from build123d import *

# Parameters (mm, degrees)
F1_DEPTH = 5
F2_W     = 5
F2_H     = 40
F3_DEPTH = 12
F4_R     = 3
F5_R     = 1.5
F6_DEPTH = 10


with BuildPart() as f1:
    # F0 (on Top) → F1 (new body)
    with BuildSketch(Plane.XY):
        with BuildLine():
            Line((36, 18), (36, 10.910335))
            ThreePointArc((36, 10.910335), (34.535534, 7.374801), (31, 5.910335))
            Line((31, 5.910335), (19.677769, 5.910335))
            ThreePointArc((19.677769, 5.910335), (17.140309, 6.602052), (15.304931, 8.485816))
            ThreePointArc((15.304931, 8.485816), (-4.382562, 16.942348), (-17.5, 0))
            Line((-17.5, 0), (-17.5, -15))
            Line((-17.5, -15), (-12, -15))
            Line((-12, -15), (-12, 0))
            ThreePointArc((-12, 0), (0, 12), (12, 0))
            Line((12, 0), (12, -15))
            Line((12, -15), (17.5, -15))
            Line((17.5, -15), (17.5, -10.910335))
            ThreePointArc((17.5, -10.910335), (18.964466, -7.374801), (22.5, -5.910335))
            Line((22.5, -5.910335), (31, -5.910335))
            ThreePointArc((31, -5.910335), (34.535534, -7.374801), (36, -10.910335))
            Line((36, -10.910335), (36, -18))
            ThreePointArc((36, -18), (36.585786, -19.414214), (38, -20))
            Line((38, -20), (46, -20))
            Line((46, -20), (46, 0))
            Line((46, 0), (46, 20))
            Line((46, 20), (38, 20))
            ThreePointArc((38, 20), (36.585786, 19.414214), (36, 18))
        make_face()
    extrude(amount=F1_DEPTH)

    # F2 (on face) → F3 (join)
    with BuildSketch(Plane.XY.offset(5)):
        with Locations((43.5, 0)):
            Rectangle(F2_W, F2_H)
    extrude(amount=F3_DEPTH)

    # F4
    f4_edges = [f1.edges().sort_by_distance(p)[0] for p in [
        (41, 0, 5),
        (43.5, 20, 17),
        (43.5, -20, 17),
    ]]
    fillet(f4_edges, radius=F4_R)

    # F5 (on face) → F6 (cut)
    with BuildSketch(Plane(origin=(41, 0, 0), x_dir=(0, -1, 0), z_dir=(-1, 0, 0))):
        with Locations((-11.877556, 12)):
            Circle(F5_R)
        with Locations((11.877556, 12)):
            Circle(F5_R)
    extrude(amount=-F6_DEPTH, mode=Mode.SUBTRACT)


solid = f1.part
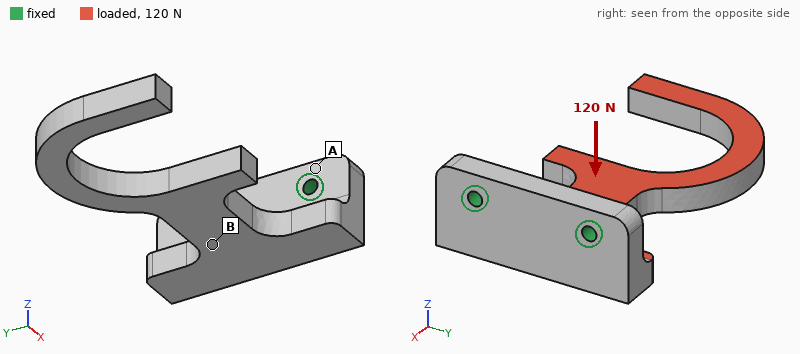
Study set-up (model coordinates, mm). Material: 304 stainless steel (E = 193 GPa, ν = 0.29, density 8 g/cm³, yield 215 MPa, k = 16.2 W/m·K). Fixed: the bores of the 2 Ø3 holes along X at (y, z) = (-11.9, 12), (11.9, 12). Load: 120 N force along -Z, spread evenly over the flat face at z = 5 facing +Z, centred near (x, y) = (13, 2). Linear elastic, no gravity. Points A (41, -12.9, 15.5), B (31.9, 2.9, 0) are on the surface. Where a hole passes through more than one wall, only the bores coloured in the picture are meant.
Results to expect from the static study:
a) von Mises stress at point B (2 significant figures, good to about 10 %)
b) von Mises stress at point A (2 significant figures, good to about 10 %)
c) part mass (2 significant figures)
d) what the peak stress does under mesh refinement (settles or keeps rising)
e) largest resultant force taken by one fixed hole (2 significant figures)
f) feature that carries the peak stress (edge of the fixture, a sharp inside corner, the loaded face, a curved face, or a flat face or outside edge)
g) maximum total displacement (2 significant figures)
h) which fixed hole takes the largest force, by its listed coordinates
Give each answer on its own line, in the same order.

45 MPa
6.8 MPa
61 g
keeps rising
78 N
edge of the fixture
0.20 mm
(11.9, 12)
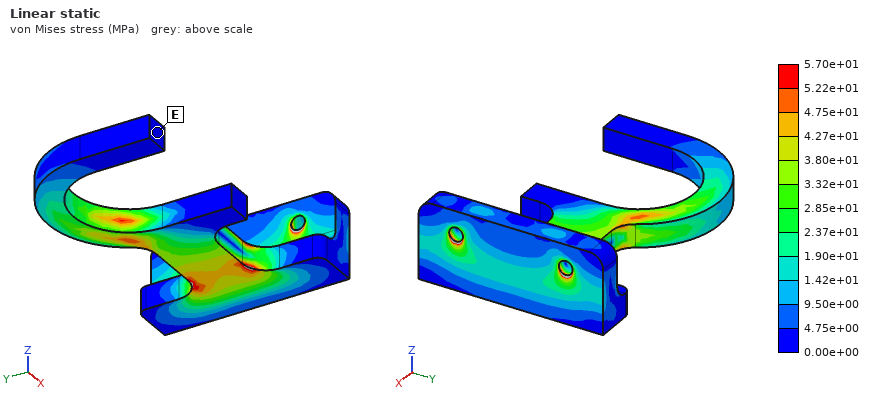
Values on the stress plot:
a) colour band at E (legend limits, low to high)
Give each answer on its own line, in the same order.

0.00e+00 to 4.75e+00 MPa
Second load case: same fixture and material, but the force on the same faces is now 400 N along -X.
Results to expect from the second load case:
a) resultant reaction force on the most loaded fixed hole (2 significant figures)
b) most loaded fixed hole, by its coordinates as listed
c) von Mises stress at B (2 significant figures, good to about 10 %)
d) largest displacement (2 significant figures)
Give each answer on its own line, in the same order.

230 N
(11.9, 12)
9.4 MPa
0.10 mm
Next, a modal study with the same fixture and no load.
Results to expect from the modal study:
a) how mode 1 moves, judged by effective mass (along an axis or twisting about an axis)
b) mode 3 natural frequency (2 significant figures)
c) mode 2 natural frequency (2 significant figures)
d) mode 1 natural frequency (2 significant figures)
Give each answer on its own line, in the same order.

along Z
2400 Hz
1500 Hz
890 Hz
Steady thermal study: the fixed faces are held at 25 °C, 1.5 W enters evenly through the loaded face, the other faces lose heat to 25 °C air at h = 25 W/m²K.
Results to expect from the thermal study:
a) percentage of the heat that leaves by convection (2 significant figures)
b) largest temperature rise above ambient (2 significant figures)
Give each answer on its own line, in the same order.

51 %
23 K
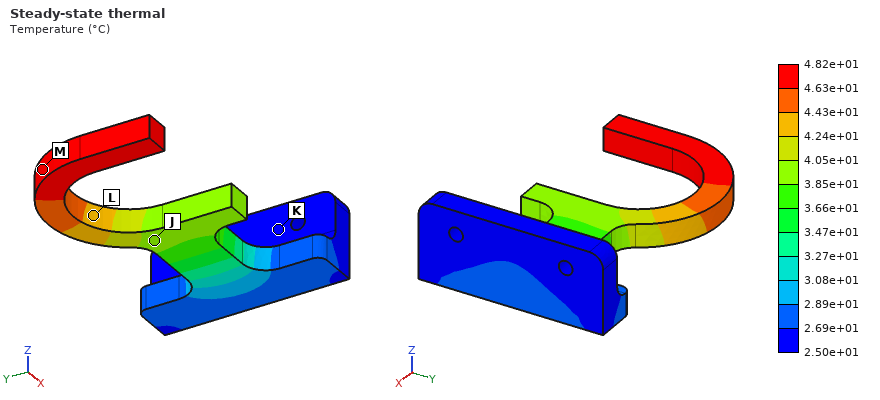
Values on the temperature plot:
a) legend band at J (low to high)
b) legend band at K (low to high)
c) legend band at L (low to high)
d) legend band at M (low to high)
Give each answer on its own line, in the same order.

3.85e+01 to 4.05e+01 °C
2.50e+01 to 2.69e+01 °C
4.24e+01 to 4.43e+01 °C
4.63e+01 to 4.82e+01 °C
